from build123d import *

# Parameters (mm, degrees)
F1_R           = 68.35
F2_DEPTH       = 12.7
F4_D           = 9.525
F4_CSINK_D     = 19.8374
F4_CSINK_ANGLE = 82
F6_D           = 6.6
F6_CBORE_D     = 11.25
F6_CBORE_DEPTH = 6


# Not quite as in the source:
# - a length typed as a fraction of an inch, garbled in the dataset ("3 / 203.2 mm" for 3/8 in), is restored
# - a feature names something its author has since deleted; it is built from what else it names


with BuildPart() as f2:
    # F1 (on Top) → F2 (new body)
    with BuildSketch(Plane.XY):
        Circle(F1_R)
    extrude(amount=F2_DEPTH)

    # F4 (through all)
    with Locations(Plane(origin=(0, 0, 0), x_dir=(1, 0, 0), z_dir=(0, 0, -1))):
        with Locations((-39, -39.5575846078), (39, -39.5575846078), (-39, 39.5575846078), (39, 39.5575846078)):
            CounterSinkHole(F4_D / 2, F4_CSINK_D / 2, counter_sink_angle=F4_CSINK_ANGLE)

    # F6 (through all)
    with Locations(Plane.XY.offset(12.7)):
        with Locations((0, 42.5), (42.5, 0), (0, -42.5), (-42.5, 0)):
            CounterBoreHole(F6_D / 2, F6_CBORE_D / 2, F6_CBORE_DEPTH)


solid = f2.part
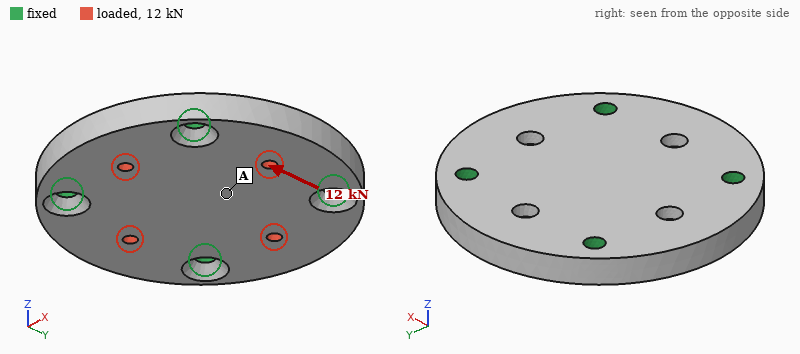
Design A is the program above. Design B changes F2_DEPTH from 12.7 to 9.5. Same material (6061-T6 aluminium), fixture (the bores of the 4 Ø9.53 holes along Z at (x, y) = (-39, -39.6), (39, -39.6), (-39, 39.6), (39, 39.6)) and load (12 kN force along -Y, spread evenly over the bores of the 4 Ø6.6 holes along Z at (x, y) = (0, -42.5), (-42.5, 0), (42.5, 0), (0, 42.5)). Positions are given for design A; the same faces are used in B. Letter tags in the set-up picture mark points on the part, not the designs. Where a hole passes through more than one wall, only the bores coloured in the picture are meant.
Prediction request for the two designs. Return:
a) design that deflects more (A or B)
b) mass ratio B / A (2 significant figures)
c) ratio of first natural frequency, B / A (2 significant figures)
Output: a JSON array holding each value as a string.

["B", "0.75", "0.76"]
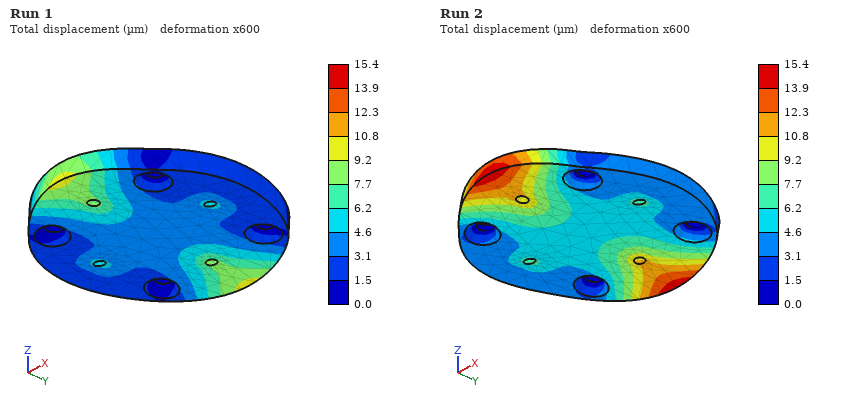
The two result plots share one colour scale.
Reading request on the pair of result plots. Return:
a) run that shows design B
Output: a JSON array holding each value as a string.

["Run 2"]
